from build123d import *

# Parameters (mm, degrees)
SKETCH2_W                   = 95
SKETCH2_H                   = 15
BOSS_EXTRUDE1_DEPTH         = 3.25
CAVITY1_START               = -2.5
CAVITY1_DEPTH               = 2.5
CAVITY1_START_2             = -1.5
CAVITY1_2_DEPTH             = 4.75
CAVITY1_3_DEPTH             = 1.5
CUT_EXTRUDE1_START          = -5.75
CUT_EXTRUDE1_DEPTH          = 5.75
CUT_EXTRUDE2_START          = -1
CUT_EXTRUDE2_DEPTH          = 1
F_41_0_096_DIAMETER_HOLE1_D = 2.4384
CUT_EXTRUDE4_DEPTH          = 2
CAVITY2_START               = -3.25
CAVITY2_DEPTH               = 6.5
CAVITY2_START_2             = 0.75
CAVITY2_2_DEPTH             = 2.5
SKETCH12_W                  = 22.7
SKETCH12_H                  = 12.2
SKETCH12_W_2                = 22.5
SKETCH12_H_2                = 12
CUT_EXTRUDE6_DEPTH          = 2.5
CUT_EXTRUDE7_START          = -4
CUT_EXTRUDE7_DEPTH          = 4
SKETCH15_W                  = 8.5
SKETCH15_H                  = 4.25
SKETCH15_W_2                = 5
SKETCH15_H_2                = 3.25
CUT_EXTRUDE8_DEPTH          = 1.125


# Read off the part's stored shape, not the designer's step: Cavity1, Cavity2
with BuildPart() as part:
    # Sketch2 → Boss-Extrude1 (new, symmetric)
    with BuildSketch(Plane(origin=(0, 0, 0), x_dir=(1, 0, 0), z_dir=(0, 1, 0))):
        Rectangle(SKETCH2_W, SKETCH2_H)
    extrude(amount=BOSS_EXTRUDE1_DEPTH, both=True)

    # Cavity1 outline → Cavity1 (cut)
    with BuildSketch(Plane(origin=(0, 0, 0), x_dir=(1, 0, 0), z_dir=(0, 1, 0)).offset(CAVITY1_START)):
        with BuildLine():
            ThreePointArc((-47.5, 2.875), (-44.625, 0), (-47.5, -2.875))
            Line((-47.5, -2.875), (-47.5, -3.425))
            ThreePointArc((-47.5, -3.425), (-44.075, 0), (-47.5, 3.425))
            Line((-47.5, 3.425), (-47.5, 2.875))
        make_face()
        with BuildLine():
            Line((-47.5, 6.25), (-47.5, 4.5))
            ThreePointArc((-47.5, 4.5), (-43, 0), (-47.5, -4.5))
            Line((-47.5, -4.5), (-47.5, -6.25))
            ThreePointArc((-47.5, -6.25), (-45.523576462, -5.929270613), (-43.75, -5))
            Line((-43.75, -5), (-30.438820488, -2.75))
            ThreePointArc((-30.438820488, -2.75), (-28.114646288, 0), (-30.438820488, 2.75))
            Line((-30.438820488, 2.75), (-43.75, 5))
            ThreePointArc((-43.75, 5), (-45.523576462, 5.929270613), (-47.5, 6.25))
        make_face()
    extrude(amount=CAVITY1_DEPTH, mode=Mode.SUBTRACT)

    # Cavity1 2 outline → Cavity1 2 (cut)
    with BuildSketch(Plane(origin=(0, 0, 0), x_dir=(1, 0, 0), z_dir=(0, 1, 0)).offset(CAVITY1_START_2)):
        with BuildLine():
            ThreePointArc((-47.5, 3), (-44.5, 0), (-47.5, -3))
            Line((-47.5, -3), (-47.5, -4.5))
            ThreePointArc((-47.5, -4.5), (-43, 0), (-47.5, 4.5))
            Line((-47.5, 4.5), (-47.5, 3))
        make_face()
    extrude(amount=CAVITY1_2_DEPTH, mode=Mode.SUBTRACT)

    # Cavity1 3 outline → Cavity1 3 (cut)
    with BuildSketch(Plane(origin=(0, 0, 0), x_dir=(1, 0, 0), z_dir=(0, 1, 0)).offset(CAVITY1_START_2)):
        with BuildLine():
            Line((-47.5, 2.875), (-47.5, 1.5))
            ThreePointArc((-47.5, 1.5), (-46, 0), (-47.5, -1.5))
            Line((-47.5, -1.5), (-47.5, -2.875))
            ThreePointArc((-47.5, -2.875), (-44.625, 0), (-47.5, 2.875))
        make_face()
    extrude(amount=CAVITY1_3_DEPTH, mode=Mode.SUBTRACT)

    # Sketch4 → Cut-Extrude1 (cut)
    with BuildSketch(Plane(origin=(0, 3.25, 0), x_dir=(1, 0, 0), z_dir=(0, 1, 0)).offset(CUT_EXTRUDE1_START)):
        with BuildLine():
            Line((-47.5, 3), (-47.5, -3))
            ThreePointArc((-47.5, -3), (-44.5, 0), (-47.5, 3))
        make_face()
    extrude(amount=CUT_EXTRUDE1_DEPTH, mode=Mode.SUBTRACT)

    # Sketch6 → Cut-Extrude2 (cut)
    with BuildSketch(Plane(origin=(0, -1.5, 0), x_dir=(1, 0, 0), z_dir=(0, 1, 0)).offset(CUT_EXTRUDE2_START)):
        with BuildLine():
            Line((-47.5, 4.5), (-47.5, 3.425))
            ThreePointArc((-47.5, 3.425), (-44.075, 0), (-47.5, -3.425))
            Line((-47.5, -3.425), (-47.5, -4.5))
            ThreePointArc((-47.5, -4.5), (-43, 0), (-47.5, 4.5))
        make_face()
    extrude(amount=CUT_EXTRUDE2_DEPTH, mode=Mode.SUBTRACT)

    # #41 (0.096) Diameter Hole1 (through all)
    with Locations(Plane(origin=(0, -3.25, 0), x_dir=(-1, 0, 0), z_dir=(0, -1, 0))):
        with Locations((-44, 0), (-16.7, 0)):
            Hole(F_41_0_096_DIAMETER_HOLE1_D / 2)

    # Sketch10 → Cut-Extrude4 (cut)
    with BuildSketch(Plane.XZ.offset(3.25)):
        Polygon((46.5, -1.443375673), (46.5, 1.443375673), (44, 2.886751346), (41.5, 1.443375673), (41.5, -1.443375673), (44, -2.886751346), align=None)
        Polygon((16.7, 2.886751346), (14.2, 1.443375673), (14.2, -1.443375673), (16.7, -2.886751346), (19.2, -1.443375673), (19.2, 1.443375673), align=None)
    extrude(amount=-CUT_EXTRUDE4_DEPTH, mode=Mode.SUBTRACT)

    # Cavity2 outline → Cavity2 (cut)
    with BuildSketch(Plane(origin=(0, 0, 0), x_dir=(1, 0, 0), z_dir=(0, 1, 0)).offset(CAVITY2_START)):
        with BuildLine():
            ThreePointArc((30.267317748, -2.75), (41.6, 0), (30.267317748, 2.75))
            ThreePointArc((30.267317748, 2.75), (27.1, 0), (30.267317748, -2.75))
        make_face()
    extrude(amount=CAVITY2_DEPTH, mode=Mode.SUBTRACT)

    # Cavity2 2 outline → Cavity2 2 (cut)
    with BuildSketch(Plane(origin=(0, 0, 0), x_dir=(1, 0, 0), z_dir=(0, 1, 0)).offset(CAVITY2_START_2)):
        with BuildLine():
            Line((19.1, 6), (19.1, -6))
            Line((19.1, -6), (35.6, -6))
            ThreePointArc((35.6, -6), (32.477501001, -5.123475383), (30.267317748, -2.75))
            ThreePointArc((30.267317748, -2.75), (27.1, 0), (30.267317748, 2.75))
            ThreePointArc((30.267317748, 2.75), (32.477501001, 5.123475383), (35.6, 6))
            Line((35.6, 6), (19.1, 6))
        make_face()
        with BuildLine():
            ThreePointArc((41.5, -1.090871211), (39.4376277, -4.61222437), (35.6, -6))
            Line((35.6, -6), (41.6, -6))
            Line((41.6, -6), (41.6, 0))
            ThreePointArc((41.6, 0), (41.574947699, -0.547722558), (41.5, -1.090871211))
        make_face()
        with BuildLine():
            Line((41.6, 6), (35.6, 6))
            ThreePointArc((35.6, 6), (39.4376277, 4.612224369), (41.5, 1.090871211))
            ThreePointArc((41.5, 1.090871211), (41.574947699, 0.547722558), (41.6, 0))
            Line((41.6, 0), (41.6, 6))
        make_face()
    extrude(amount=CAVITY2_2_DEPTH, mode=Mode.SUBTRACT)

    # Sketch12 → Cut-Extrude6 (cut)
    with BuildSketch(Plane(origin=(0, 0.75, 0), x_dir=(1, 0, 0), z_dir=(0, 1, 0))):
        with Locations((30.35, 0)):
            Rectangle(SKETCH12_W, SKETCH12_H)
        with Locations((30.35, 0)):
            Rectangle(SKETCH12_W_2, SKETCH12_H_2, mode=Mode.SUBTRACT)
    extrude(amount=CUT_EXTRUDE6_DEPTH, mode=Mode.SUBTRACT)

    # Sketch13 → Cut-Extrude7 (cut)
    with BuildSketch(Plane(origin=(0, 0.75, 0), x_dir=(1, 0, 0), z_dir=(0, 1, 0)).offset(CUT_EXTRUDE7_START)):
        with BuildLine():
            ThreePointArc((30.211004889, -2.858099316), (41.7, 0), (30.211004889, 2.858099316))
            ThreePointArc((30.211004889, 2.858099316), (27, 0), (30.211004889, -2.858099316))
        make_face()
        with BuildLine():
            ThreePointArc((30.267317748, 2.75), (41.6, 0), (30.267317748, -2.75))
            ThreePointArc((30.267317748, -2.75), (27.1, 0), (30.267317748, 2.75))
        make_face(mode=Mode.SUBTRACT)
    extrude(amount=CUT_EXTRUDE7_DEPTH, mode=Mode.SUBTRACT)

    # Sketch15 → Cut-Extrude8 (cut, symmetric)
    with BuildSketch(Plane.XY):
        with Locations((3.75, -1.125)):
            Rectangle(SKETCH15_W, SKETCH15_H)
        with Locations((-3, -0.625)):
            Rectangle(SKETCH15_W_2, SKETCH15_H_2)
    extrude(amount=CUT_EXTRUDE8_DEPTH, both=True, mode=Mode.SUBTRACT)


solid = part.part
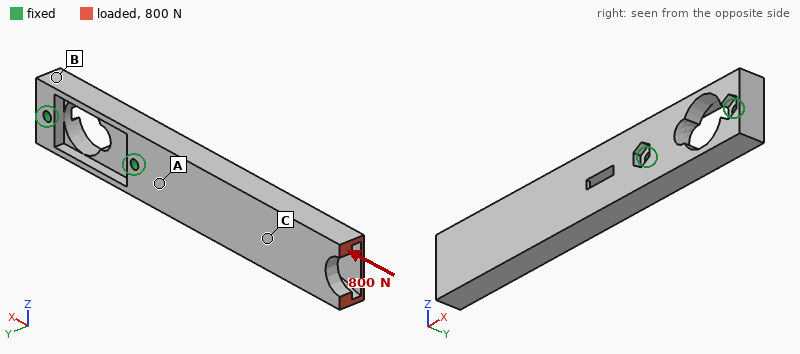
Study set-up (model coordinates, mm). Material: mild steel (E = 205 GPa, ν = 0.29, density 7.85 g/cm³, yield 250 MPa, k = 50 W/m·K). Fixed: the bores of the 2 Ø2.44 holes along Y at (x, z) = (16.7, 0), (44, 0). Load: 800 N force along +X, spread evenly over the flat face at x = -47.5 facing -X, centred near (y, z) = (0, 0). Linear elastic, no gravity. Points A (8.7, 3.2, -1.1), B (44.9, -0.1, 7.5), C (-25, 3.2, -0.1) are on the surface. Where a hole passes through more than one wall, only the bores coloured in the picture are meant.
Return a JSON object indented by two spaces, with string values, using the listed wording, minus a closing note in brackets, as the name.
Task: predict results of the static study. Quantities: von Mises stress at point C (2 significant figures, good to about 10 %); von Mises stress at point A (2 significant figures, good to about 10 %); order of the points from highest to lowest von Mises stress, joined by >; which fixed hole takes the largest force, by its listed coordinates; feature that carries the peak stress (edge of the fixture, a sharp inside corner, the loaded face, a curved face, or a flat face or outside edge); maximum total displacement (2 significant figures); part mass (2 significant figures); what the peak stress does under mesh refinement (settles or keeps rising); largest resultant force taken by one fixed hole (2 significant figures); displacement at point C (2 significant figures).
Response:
{
  "von Mises stress at point C": "6.0 MPa",
  "von Mises stress at point A": "8.9 MPa",
  "order of the points from highest to lowest von Mises stress, joined by >": "A > C > B",
  "which fixed hole takes the largest force, by its listed coordinates": "(16.7, 0)",
  "feature that carries the peak stress": "edge of the fixture",
  "maximum total displacement": "14 µm",
  "part mass": "57 g",
  "what the peak stress does under mesh refinement": "keeps rising",
  "largest resultant force taken by one fixed hole": "750 N",
  "displacement at point C": "6.8 µm"
}
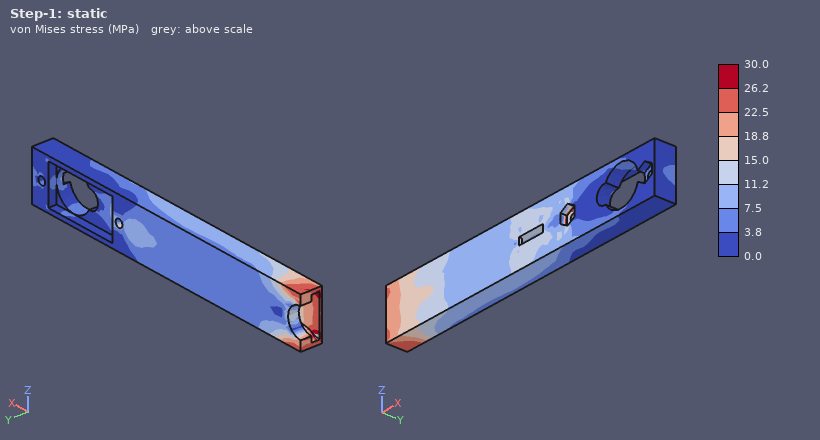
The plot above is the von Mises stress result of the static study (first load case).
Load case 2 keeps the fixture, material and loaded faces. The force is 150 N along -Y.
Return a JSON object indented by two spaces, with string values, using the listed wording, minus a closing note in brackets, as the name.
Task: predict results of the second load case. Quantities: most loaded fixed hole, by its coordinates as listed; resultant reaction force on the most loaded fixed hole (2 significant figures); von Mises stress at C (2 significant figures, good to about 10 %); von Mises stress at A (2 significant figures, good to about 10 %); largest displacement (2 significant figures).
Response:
{
  "most loaded fixed hole, by its coordinates as listed": "(16.7, 0)",
  "resultant reaction force on the most loaded fixed hole": "310 N",
  "von Mises stress at C": "32 MPa",
  "von Mises stress at A": "83 MPa",
  "largest displacement": "0.25 mm"
}
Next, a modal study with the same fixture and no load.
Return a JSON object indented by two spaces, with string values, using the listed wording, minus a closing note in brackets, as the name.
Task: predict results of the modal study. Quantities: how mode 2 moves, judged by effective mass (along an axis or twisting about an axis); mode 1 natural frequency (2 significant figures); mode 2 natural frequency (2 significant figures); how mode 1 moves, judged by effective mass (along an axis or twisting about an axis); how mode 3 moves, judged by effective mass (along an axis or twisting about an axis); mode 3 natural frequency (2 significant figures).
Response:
{
  "how mode 2 moves, judged by effective mass": "along Z",
  "mode 1 natural frequency": "1300 Hz",
  "mode 2 natural frequency": "2100 Hz",
  "how mode 1 moves, judged by effective mass": "along Y",
  "how mode 3 moves, judged by effective mass": "twisting about X",
  "mode 3 natural frequency": "7400 Hz"
}
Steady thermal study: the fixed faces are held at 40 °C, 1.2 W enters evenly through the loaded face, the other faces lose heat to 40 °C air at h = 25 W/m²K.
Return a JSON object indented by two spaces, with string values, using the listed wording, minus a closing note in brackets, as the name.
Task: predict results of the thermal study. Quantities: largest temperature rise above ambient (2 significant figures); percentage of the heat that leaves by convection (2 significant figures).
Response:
{
  "largest temperature rise above ambient": "14 K",
  "percentage of the heat that leaves by convection": "43 %"
}
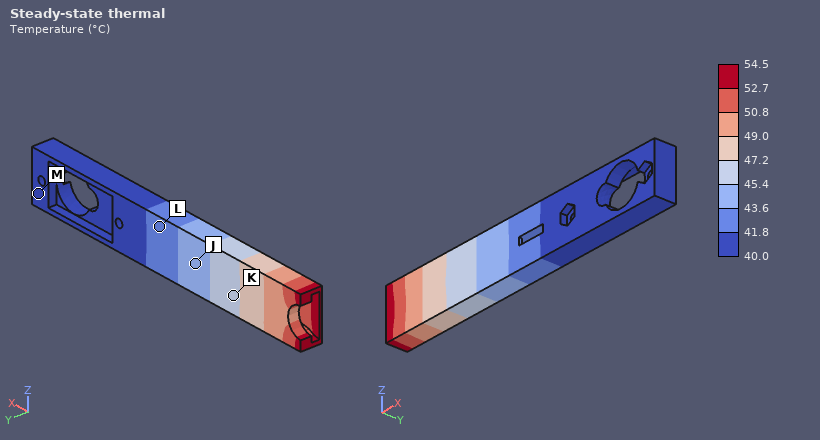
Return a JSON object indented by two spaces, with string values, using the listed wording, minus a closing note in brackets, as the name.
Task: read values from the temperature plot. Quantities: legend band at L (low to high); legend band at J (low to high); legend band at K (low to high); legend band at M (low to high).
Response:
{
  "legend band at L": "41.8 to 43.6 °C",
  "legend band at J": "43.6 to 45.4 °C",
  "legend band at K": "45.4 to 47.2 °C",
  "legend band at M": "40.0 to 41.8 °C"
}
